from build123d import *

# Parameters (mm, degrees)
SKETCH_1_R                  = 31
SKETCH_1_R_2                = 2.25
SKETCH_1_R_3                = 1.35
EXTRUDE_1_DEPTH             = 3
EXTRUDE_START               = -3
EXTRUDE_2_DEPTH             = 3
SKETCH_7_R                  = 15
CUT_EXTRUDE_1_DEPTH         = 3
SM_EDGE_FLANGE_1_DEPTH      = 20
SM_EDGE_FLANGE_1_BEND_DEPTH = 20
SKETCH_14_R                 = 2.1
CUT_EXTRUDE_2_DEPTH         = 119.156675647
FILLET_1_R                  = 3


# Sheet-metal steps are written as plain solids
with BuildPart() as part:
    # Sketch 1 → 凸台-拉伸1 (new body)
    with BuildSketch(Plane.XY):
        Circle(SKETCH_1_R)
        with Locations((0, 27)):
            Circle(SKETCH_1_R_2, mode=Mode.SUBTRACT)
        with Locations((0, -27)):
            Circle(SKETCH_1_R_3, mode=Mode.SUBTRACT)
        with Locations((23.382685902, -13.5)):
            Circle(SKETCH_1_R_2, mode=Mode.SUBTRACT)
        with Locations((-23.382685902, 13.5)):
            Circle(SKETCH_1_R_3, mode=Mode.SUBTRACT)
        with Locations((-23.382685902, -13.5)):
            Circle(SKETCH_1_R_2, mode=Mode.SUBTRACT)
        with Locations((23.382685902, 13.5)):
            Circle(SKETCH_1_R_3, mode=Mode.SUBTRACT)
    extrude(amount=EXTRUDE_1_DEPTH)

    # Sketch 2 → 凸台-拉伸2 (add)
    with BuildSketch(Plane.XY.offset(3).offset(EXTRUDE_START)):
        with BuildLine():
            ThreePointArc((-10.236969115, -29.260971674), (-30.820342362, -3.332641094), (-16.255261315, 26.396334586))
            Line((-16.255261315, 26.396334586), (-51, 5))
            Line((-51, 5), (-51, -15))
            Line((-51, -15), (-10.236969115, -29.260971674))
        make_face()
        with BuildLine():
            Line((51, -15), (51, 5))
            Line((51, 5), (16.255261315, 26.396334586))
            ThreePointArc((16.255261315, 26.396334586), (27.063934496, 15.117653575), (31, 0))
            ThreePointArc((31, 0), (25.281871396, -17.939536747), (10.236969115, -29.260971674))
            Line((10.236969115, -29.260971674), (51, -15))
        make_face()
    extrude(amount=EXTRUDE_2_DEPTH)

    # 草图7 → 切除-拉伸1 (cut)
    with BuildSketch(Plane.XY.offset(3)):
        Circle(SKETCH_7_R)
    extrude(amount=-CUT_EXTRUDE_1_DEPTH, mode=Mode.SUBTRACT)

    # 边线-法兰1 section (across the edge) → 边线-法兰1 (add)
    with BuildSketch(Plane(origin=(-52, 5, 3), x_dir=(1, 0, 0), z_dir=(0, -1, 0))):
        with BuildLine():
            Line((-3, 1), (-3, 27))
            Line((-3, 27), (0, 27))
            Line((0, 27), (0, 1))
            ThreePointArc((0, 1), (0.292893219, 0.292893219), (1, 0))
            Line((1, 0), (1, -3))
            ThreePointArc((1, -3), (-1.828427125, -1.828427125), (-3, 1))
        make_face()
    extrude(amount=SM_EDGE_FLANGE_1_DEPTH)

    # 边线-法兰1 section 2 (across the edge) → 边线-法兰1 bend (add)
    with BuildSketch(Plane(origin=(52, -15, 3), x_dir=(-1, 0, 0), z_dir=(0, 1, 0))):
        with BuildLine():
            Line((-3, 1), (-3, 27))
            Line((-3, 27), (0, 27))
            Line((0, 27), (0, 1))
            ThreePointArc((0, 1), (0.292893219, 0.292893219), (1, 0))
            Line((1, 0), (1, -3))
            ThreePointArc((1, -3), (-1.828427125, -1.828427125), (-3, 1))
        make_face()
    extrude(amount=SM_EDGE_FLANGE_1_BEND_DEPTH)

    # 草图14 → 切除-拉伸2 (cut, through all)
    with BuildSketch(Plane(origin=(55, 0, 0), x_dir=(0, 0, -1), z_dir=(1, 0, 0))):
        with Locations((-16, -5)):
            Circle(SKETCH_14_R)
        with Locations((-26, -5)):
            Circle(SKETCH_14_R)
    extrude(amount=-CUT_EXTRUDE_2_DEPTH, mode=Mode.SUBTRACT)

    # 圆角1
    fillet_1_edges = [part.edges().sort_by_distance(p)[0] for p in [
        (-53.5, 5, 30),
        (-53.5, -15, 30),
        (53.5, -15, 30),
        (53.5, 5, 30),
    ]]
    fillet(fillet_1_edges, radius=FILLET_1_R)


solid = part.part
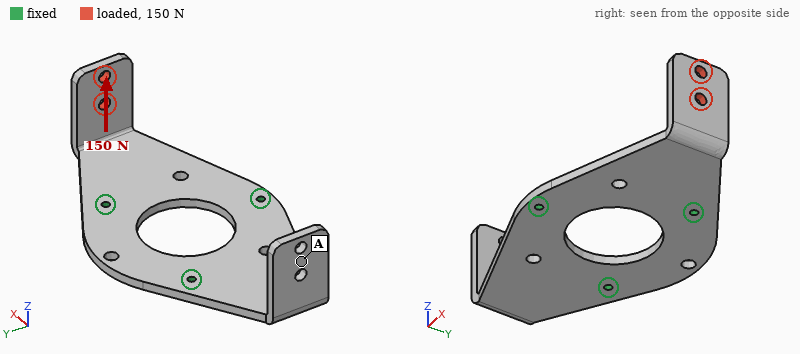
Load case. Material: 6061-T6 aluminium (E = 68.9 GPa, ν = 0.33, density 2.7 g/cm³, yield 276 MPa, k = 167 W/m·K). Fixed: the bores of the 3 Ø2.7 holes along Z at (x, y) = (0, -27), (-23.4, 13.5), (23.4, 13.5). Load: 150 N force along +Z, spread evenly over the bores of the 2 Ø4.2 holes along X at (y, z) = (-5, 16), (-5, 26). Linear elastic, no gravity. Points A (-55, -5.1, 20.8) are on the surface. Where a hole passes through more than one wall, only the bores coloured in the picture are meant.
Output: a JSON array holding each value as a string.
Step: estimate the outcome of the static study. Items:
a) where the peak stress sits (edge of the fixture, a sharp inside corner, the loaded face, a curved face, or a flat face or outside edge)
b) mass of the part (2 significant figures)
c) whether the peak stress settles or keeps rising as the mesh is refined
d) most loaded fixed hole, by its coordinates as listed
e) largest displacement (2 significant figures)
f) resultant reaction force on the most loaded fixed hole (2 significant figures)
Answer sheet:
["edge of the fixture", "39 g", "keeps rising", "(23.4, 13.5)", "0.83 mm", "160 N"]
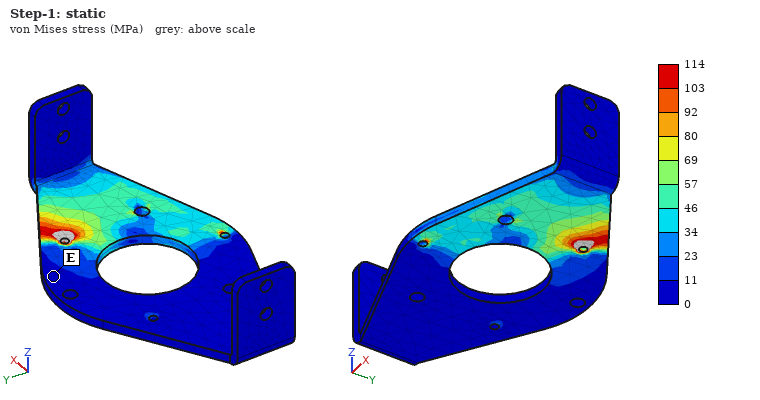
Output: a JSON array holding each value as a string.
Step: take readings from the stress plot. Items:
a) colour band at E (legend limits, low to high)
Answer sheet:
["0 to 11 MPa"]
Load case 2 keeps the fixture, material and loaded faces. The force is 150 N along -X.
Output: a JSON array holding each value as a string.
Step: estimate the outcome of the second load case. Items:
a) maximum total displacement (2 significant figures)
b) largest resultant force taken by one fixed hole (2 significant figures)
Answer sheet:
["0.93 mm", "86 N"]
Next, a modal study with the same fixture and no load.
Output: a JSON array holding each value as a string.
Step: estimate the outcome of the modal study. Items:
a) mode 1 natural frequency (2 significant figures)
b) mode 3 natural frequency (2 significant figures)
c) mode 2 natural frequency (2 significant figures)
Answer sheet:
["940 Hz", "1900 Hz", "950 Hz"]
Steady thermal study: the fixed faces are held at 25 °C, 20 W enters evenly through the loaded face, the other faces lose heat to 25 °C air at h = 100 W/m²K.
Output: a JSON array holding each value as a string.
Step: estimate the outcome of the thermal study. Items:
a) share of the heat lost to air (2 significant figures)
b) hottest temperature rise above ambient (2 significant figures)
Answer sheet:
["52 %", "65 K"]
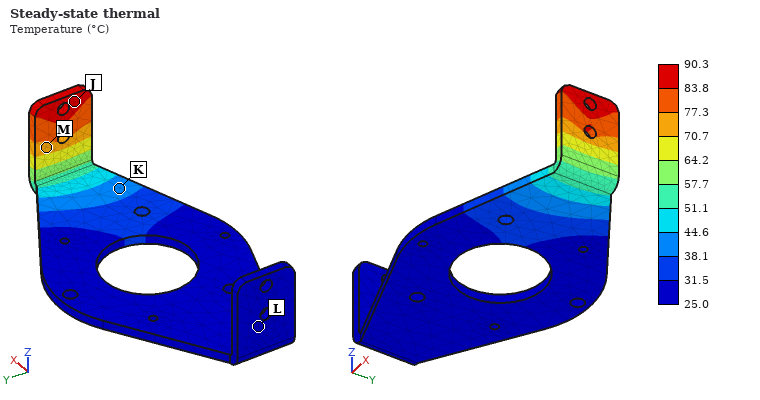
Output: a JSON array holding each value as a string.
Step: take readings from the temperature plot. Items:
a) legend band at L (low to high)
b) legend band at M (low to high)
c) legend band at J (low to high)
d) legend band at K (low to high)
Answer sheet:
["25.0 to 31.5 °C", "70.7 to 77.3 °C", "83.8 to 90.3 °C", "38.1 to 44.6 °C"]
